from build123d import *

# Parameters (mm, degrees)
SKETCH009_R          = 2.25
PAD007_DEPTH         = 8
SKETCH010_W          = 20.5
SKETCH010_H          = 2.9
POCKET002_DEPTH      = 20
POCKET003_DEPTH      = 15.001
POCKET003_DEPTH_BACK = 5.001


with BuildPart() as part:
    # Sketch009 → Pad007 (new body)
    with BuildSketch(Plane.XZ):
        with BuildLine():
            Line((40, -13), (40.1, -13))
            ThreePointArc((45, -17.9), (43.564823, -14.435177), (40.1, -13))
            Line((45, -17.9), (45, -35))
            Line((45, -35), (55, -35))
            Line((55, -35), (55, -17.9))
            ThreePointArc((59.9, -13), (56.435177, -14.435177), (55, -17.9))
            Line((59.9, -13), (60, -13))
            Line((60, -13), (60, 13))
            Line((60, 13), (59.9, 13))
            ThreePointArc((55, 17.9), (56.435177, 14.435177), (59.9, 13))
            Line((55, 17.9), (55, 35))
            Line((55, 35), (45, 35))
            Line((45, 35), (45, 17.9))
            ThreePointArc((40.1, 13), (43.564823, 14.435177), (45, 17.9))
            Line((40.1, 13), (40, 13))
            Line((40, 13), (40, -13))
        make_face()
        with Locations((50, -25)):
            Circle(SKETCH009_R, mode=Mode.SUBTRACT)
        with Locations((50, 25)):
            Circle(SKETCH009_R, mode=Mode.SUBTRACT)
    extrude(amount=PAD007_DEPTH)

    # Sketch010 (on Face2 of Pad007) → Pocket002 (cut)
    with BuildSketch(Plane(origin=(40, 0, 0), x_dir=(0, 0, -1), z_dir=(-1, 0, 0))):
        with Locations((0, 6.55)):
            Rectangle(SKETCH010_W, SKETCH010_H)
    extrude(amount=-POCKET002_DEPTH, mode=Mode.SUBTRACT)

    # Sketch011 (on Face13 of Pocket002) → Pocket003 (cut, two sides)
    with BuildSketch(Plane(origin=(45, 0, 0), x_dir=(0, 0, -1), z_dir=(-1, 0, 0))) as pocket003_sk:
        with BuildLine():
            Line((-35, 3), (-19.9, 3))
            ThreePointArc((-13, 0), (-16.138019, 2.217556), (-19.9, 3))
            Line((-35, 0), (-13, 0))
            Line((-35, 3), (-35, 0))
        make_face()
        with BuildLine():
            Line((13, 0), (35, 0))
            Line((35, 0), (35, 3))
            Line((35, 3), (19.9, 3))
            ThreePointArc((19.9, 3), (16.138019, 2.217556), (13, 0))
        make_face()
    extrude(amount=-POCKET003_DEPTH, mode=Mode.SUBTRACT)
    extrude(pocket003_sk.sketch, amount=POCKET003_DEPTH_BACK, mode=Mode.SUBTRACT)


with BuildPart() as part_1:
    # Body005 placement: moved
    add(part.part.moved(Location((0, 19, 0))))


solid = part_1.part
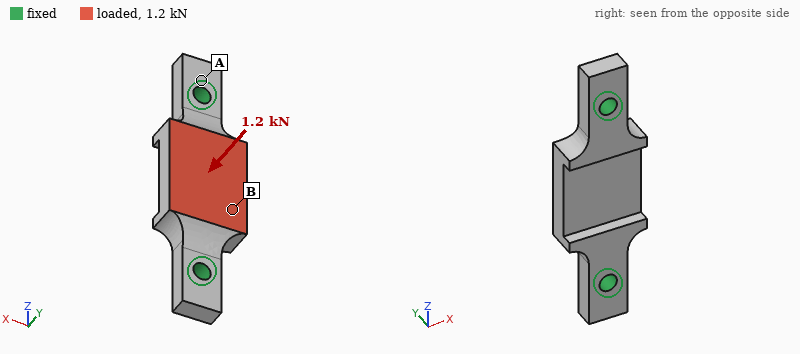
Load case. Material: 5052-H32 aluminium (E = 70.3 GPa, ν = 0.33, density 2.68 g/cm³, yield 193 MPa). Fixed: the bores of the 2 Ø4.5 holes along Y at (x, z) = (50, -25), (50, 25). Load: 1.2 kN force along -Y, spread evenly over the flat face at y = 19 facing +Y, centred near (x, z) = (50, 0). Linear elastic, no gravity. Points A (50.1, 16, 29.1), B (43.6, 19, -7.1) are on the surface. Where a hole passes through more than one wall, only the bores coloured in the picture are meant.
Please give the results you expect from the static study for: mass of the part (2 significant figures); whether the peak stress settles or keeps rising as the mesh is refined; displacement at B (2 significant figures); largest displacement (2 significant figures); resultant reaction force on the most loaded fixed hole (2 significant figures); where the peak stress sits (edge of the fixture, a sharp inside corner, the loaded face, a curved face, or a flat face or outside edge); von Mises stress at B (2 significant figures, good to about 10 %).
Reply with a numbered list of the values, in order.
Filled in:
1. 14 g
2. keeps rising
3. 31 µm
4. 37 µm
5. 1.2 kN
6. edge of the fixture
7. 33 MPa
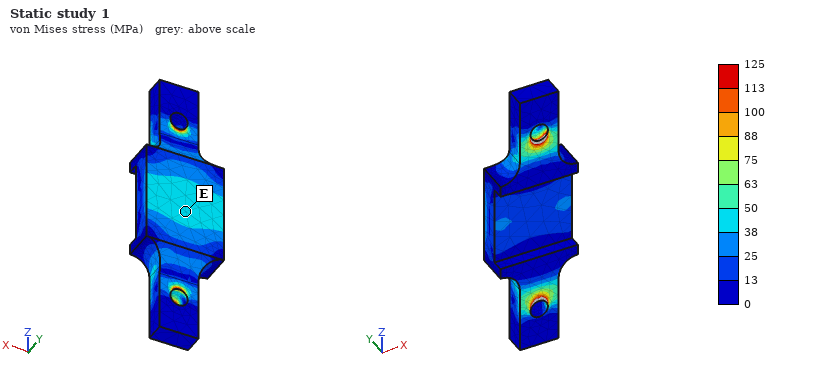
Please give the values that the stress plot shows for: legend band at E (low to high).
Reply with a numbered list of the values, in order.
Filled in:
1. 38 to 50 MPa
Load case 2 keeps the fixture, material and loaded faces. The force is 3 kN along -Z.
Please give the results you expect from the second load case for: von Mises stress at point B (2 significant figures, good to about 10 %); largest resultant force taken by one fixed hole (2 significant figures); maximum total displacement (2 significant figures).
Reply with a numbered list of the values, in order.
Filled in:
1. 12 MPa
2. 1.6 kN
3. 9.0 µm
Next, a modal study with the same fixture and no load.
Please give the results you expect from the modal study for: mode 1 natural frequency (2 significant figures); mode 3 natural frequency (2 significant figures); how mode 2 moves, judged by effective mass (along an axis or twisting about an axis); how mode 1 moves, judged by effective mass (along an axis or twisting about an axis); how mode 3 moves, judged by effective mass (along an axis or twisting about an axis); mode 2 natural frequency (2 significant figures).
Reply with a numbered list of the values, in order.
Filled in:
1. 10 kHz
2. 19 kHz
3. along Y
4. along X
5. along X
6. 11 kHz
